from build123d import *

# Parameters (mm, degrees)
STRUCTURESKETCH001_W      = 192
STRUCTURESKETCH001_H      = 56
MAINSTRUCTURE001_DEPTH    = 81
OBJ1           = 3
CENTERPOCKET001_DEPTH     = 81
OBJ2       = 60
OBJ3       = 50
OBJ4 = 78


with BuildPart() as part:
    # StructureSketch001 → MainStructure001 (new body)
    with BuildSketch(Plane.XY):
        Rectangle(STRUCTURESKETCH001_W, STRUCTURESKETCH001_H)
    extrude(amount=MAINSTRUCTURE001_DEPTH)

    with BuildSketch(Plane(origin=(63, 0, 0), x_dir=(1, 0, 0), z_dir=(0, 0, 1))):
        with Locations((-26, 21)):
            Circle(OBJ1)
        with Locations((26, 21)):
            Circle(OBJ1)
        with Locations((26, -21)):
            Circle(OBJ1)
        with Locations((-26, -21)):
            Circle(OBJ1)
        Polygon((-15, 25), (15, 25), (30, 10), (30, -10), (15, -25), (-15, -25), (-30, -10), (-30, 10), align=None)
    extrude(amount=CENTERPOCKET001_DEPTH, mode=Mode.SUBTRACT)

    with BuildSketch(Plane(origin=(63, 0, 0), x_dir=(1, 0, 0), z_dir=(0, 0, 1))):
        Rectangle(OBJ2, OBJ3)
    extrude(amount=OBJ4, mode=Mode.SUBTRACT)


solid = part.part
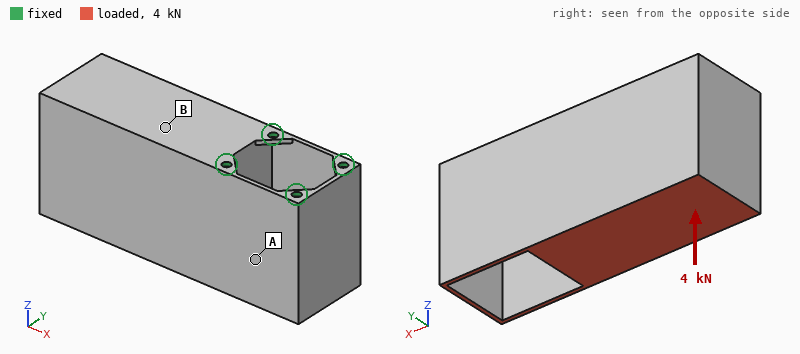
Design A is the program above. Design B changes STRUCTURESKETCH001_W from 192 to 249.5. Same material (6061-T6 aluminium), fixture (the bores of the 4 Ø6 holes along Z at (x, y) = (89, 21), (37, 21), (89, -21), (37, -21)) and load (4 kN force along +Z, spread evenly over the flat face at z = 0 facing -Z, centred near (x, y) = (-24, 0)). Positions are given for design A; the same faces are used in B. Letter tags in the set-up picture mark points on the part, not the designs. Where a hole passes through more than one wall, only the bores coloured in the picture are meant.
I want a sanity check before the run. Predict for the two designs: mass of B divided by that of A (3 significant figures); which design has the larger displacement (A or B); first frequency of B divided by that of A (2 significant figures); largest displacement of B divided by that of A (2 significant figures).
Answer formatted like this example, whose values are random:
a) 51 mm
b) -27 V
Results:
a) 1.41
b) B
c) 0.79
d) 1.1
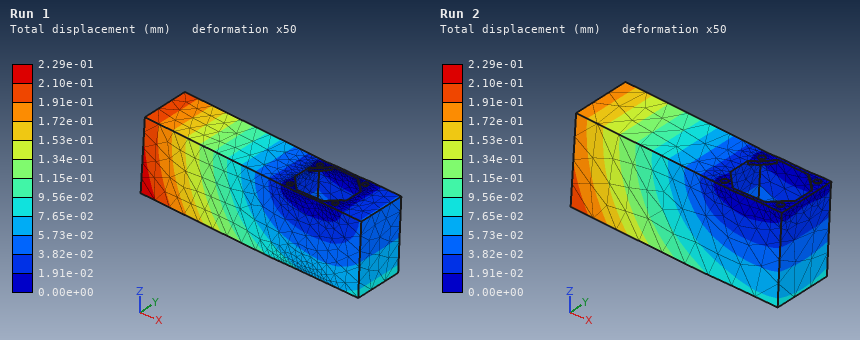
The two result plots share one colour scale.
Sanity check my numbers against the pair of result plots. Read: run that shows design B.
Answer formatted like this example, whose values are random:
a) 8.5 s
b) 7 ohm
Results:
a) Run 1
